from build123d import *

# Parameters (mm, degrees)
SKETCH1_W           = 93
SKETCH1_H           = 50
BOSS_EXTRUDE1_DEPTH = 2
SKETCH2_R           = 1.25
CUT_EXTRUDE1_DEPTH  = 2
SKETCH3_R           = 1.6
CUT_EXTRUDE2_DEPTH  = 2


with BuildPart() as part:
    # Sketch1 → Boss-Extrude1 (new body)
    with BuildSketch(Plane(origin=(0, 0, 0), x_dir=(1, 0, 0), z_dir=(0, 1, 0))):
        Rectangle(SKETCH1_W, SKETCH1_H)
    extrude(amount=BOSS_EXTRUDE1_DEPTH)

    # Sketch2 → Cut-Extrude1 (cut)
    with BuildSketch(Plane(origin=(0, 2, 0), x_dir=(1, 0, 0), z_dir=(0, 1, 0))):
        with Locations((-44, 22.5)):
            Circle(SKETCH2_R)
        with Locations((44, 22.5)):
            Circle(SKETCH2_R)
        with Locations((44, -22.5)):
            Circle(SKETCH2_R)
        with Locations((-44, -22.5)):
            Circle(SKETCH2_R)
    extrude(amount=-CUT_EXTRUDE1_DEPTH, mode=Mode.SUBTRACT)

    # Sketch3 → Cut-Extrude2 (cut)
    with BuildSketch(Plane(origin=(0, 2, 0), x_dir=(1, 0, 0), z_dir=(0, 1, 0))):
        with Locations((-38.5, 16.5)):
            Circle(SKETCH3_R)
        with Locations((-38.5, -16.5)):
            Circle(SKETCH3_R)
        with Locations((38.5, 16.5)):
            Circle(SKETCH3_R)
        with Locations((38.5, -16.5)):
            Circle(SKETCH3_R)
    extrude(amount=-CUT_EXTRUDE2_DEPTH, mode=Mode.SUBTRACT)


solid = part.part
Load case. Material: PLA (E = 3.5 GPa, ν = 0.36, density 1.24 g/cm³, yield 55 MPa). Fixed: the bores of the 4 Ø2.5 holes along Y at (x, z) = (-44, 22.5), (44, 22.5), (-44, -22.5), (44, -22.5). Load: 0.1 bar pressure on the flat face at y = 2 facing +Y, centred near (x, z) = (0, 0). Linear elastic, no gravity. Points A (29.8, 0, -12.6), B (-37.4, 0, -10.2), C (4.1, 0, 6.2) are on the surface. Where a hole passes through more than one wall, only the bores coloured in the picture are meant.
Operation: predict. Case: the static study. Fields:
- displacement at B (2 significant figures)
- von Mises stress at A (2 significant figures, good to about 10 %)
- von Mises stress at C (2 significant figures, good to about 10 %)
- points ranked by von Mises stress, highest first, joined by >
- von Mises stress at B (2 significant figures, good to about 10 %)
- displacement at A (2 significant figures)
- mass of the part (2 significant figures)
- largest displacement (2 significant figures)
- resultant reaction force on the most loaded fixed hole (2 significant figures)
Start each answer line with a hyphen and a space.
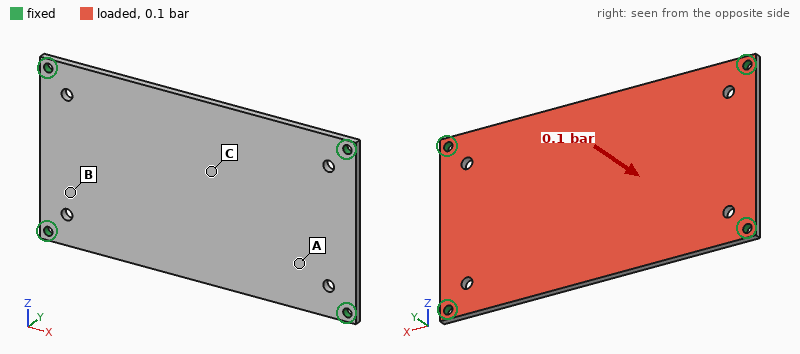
- 0.20 mm
- 1.9 MPa
- 5.4 MPa
- C > B > A
- 3.2 MPa
- 0.41 mm
- 11 g
- 1.0 mm
- 11 N
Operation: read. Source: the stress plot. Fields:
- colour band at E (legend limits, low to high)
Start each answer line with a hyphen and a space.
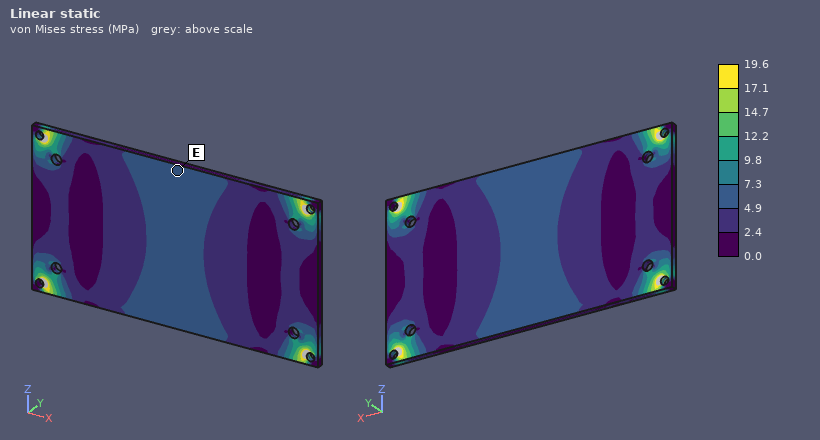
- 4.9 to 7.3 MPa
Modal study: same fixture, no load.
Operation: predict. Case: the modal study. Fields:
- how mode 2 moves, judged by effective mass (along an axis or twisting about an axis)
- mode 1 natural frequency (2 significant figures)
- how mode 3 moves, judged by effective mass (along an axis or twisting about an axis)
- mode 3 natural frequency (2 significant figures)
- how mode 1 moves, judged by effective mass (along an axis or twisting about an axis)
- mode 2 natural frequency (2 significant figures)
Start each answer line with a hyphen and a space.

- twisting about X
- 360 Hz
- twisting about Z
- 1000 Hz
- along Y
- 660 Hz
